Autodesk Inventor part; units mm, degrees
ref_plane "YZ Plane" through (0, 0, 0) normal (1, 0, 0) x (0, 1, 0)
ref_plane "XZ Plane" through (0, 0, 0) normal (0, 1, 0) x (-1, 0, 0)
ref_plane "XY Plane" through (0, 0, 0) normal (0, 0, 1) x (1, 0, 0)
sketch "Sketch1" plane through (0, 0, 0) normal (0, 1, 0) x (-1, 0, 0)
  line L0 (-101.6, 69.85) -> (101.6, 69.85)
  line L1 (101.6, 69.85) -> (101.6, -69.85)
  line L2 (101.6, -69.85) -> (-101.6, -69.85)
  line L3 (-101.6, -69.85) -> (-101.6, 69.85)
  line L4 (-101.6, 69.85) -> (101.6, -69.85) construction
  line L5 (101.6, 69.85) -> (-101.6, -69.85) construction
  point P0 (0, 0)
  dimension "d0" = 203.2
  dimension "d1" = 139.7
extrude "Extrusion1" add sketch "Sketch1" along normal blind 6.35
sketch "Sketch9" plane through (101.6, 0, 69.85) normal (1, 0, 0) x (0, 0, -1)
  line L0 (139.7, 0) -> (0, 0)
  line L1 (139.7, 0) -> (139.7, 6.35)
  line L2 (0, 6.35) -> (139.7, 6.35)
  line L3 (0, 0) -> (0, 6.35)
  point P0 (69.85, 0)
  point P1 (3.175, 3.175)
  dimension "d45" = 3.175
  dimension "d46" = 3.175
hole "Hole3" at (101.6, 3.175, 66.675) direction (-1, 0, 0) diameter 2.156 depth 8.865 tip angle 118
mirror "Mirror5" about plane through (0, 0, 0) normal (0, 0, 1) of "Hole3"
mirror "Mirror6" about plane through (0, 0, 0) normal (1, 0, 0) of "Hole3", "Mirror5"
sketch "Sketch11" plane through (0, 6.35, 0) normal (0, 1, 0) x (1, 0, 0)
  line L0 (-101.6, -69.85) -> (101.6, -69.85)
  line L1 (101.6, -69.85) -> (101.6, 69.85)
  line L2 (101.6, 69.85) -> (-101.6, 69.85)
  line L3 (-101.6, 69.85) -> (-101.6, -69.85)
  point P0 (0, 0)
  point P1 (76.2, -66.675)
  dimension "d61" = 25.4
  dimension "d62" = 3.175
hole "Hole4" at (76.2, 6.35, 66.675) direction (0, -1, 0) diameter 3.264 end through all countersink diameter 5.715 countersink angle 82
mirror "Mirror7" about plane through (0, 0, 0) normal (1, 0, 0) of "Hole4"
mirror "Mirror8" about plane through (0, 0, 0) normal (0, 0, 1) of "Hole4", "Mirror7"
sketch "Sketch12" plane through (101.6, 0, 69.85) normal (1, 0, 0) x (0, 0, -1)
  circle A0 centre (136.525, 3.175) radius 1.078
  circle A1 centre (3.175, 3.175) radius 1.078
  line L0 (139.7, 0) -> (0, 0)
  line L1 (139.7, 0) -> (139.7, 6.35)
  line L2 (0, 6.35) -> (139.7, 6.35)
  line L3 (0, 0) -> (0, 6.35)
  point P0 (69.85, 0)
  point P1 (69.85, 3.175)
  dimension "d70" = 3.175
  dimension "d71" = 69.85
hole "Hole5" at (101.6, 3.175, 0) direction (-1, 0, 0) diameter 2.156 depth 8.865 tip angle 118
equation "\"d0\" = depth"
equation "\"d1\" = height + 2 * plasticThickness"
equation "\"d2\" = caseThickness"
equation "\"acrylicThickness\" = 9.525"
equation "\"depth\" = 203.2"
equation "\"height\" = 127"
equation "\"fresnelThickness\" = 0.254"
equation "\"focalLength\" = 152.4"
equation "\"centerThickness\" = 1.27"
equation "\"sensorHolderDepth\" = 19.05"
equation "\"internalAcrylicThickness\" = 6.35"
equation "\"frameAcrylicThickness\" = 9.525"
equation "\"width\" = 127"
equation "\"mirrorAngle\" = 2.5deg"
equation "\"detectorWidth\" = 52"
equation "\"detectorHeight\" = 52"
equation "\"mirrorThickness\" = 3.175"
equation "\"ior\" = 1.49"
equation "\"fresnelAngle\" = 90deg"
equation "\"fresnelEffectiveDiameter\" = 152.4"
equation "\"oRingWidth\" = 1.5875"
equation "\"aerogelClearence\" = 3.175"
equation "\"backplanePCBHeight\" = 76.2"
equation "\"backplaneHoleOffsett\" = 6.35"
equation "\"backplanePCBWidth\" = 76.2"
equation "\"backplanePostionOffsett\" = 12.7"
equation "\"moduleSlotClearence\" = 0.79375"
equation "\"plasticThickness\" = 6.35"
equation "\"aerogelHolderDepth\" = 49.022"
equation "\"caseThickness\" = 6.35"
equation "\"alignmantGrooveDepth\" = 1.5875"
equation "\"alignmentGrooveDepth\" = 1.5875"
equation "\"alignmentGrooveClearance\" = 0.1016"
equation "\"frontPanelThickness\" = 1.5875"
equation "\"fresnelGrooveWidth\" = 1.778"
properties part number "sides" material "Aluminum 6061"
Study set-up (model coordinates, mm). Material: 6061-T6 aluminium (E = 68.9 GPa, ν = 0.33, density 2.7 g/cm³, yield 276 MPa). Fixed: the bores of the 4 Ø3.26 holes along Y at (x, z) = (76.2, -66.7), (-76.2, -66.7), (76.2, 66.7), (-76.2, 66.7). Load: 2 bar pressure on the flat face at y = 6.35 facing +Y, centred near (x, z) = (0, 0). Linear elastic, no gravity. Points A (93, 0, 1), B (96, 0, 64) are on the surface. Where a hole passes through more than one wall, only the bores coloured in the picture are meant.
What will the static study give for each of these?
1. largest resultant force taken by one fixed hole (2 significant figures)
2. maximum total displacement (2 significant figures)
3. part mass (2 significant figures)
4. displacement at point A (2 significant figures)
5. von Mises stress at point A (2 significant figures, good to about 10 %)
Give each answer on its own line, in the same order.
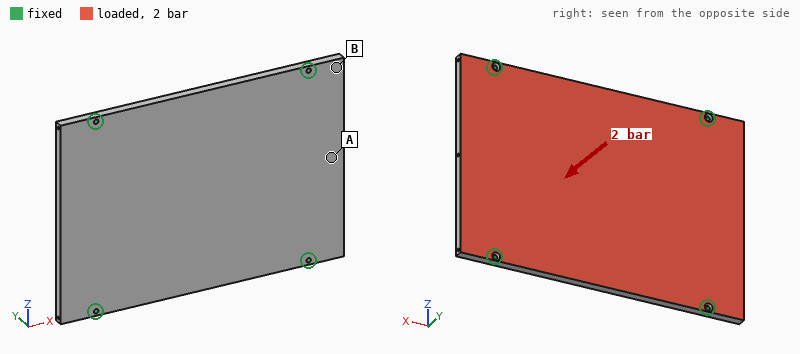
1.5 kN
0.57 mm
490 g
0.22 mm
39 MPa
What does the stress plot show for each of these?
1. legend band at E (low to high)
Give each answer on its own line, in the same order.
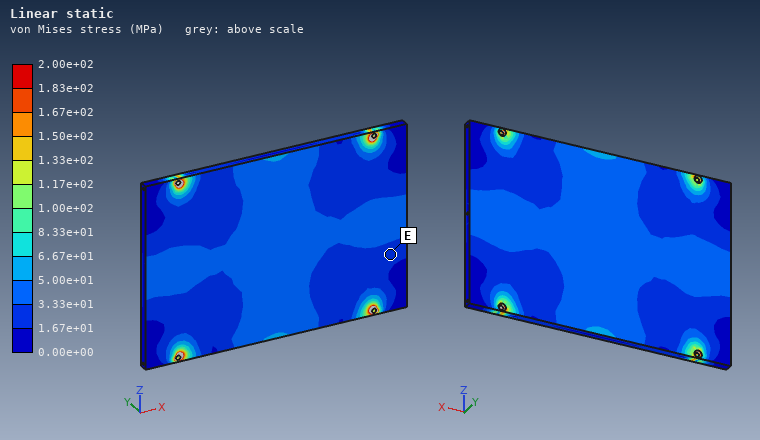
1.67e+01 to 3.33e+01 MPa
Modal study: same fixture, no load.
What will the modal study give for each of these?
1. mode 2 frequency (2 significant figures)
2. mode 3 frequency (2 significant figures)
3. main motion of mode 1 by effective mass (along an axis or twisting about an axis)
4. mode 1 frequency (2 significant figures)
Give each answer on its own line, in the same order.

1500 Hz
1500 Hz
along Y
840 Hz
